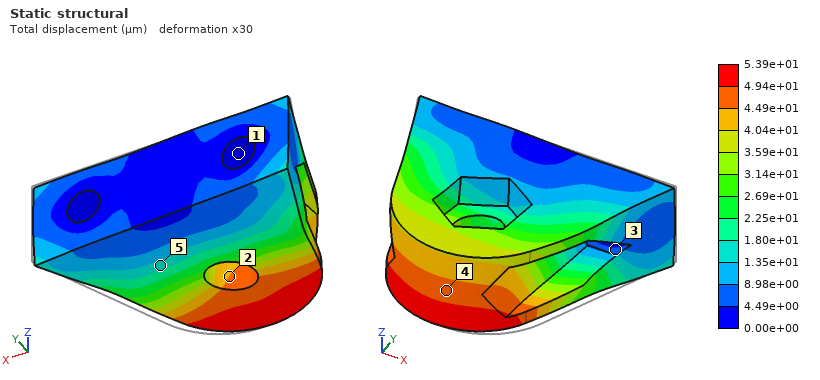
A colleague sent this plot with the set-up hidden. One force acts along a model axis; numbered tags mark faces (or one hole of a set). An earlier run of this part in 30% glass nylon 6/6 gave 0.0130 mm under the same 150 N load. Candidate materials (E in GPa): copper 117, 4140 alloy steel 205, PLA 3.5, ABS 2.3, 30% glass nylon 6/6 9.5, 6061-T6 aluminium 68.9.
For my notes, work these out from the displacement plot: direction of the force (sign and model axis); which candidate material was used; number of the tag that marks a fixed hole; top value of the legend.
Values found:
-X
ABS
1
5.39e+01 µm
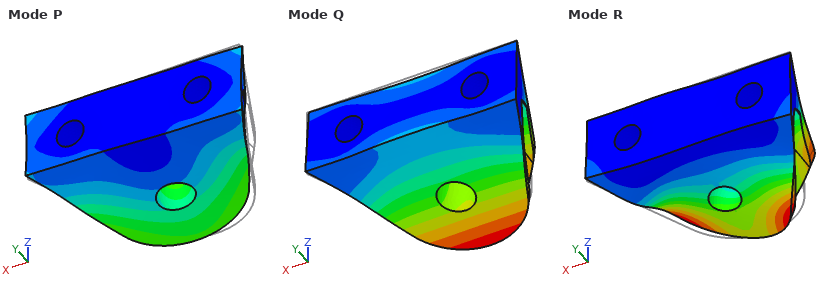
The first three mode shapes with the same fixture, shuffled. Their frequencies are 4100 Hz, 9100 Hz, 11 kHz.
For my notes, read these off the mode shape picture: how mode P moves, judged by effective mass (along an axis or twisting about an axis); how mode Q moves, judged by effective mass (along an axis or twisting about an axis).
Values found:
along X
along Z
